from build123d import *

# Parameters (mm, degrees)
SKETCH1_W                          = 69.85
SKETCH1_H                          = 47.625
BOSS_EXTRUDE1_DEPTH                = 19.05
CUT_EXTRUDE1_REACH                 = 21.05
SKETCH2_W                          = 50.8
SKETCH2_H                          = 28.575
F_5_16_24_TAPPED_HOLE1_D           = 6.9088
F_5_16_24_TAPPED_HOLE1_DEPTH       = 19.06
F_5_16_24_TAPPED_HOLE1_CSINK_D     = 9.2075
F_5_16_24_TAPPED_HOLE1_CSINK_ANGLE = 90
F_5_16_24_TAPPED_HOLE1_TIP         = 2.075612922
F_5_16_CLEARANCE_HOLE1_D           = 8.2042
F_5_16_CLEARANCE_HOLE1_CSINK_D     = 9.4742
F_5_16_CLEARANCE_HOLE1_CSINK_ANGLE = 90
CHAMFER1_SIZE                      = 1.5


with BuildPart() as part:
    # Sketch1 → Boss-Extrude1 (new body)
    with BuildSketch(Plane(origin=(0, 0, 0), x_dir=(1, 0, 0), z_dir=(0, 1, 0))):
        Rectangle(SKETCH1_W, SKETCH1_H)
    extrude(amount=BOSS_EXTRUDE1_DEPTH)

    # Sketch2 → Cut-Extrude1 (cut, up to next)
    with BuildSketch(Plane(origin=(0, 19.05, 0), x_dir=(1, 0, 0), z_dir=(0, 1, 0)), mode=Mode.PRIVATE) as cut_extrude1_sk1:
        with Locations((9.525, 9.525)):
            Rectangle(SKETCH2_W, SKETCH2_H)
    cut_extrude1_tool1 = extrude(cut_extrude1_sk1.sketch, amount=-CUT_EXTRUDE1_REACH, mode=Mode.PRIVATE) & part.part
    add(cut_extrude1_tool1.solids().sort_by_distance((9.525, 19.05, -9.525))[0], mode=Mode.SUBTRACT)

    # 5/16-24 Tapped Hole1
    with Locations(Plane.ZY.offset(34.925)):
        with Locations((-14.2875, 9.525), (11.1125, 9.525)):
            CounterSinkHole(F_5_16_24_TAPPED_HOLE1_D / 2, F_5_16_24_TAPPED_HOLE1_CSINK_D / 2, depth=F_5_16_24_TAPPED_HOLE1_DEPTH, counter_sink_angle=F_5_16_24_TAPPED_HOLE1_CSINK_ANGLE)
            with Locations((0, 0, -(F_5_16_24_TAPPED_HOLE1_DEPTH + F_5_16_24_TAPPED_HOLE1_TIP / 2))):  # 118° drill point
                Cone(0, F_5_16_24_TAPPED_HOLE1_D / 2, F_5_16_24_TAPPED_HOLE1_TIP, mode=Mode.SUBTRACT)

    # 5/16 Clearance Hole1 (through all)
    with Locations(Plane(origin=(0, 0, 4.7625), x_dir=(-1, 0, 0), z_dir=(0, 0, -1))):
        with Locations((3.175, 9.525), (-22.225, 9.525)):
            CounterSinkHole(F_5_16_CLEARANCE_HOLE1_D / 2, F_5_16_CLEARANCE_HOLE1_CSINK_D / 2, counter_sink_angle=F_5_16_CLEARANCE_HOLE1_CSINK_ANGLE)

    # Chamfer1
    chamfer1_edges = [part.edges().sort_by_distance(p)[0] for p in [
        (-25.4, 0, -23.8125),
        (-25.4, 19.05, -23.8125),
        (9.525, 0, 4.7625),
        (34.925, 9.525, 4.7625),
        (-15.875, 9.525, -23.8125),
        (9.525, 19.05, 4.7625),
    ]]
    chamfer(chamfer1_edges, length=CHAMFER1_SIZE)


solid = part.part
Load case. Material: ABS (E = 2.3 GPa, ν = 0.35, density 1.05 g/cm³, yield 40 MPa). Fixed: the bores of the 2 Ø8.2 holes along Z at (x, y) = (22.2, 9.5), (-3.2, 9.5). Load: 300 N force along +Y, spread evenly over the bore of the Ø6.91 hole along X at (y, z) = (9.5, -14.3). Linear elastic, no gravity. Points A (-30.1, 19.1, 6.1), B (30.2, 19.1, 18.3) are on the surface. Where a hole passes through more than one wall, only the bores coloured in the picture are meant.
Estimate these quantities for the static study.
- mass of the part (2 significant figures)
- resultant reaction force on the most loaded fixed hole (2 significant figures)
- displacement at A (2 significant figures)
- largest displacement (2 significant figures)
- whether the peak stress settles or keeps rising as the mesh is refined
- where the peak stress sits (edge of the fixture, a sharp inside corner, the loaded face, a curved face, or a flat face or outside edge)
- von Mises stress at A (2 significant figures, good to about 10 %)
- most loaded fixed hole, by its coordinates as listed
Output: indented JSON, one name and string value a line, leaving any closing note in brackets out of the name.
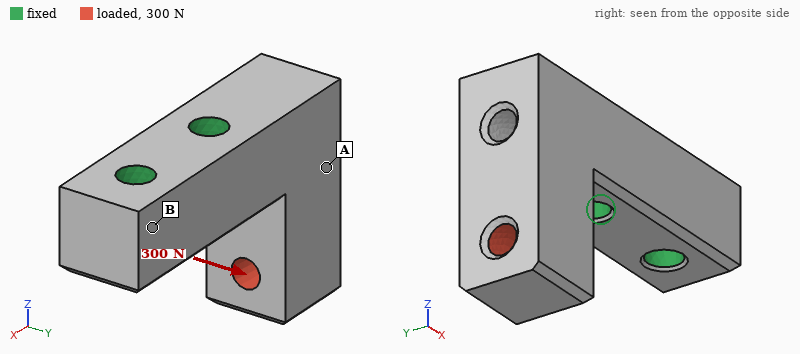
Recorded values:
{
  "mass of the part": "34 g",
  "resultant reaction force on the most loaded fixed hole": "370 N",
  "displacement at A": "0.19 mm",
  "largest displacement": "0.55 mm",
  "whether the peak stress settles or keeps rising as the mesh is refined": "keeps rising",
  "where the peak stress sits": "edge of the fixture",
  "von Mises stress at A": "3.6 MPa",
  "most loaded fixed hole, by its coordinates as listed": "(-3.2, 9.5)"
}
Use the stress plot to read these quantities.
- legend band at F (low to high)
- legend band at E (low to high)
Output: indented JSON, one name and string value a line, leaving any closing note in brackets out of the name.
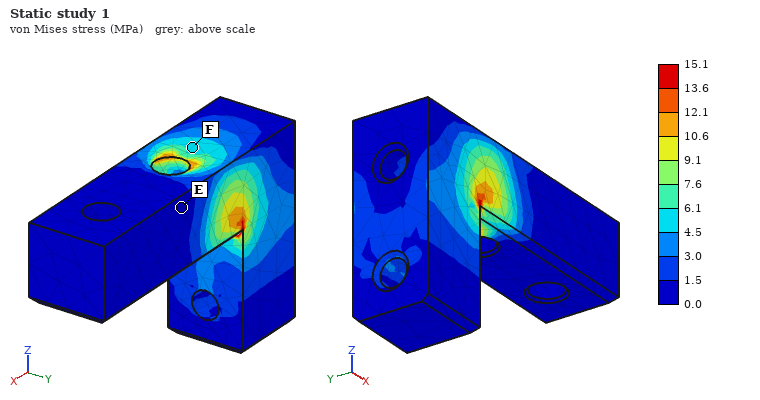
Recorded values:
{
  "legend band at F": "4.5 to 6.1 MPa",
  "legend band at E": "0.0 to 1.5 MPa"
}
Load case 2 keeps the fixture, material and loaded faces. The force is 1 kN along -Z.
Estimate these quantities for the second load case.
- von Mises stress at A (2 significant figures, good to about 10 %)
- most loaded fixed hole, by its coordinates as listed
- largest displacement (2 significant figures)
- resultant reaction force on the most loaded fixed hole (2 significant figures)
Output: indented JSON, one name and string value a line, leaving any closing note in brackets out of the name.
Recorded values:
{
  "von Mises stress at A": "3.4 MPa",
  "most loaded fixed hole, by its coordinates as listed": "(-3.2, 9.5)",
  "largest displacement": "0.50 mm",
  "resultant reaction force on the most loaded fixed hole": "1.1 kN"
}
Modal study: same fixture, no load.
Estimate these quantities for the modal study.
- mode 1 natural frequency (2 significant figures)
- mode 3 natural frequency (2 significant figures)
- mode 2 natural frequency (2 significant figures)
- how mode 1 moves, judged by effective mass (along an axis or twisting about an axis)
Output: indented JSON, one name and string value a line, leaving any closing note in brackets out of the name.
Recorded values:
{
  "mode 1 natural frequency": "1500 Hz",
  "mode 3 natural frequency": "3100 Hz",
  "mode 2 natural frequency": "1600 Hz",
  "how mode 1 moves, judged by effective mass": "along Y"
}
